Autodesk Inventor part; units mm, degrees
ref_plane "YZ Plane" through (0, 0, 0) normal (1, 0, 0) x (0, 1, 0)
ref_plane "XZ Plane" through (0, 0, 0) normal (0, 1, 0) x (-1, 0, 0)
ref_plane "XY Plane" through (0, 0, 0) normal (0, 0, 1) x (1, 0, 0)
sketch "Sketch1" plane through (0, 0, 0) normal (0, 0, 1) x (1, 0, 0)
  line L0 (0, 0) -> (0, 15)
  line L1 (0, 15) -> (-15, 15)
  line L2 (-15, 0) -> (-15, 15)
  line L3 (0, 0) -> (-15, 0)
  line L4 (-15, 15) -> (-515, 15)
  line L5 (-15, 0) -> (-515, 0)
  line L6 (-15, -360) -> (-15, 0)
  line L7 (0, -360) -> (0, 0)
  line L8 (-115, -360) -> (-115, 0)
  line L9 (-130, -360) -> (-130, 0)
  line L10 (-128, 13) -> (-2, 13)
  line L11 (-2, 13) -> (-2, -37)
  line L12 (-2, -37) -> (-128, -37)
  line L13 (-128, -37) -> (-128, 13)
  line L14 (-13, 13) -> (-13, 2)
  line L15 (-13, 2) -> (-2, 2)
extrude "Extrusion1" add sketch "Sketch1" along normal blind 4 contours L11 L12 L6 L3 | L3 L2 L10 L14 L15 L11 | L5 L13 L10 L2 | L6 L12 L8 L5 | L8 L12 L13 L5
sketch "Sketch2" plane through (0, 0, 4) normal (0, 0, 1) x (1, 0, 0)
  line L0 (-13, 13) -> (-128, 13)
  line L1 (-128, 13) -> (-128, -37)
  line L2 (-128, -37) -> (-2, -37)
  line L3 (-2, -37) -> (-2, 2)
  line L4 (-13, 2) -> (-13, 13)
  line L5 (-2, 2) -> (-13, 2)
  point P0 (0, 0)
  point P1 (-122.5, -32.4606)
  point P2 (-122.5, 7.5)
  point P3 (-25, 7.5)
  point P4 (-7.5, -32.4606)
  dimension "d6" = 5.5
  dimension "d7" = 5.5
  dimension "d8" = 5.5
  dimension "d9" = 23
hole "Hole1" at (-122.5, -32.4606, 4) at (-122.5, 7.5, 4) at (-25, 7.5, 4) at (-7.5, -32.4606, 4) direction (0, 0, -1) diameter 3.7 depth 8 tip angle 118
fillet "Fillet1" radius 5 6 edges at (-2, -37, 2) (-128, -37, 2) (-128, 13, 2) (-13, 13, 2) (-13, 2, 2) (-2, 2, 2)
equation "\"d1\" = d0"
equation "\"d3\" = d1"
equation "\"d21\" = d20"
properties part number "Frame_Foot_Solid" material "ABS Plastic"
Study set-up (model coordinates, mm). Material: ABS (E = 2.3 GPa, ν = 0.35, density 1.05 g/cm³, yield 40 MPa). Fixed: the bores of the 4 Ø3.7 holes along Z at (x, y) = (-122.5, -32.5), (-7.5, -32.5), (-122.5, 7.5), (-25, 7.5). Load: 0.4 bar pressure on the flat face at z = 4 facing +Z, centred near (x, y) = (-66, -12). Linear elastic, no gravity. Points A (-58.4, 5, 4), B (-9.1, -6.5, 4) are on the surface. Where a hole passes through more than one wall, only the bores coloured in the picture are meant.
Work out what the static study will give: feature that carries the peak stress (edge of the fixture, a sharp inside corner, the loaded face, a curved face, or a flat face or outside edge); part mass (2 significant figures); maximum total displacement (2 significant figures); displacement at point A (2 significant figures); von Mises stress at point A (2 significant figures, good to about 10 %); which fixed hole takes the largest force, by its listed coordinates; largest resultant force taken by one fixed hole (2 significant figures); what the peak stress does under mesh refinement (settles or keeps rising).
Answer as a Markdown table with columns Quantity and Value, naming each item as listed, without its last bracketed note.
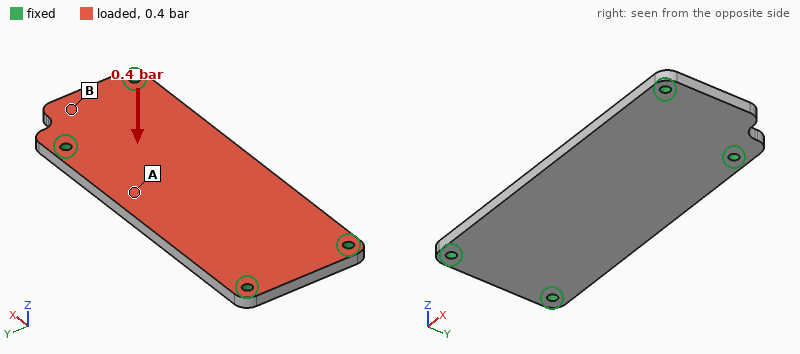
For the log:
| Quantity | Value |
|---|---|
| feature that carries the peak stress | edge of the fixture |
| part mass | 26 g |
| maximum total displacement | 1.5 mm |
| displacement at point A | 0.85 mm |
| von Mises stress at point A | 5.7 MPa |
| which fixed hole takes the largest force, by its listed coordinates | (-25, 7.5) |
| largest resultant force taken by one fixed hole | 87 N |
| what the peak stress does under mesh refinement | keeps rising |
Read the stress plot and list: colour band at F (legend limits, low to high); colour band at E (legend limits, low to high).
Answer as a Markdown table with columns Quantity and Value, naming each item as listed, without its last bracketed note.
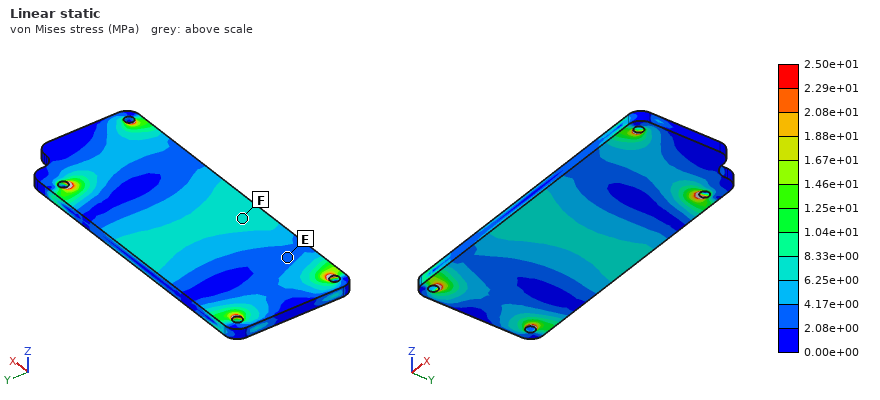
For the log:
| Quantity | Value |
|---|---|
| colour band at F | 6.25e+00 to 8.33e+00 MPa |
| colour band at E | 2.08e+00 to 4.17e+00 MPa |
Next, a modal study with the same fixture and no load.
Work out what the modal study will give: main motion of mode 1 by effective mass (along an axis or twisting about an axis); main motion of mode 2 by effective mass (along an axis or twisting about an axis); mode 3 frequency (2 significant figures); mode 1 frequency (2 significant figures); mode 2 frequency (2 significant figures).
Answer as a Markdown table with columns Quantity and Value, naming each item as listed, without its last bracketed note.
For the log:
| Quantity | Value |
|---|---|
| main motion of mode 1 by effective mass | along Z |
| main motion of mode 2 by effective mass | twisting about X |
| mode 3 frequency | 1400 Hz |
| mode 1 frequency | 510 Hz |
| mode 2 frequency | 910 Hz |
